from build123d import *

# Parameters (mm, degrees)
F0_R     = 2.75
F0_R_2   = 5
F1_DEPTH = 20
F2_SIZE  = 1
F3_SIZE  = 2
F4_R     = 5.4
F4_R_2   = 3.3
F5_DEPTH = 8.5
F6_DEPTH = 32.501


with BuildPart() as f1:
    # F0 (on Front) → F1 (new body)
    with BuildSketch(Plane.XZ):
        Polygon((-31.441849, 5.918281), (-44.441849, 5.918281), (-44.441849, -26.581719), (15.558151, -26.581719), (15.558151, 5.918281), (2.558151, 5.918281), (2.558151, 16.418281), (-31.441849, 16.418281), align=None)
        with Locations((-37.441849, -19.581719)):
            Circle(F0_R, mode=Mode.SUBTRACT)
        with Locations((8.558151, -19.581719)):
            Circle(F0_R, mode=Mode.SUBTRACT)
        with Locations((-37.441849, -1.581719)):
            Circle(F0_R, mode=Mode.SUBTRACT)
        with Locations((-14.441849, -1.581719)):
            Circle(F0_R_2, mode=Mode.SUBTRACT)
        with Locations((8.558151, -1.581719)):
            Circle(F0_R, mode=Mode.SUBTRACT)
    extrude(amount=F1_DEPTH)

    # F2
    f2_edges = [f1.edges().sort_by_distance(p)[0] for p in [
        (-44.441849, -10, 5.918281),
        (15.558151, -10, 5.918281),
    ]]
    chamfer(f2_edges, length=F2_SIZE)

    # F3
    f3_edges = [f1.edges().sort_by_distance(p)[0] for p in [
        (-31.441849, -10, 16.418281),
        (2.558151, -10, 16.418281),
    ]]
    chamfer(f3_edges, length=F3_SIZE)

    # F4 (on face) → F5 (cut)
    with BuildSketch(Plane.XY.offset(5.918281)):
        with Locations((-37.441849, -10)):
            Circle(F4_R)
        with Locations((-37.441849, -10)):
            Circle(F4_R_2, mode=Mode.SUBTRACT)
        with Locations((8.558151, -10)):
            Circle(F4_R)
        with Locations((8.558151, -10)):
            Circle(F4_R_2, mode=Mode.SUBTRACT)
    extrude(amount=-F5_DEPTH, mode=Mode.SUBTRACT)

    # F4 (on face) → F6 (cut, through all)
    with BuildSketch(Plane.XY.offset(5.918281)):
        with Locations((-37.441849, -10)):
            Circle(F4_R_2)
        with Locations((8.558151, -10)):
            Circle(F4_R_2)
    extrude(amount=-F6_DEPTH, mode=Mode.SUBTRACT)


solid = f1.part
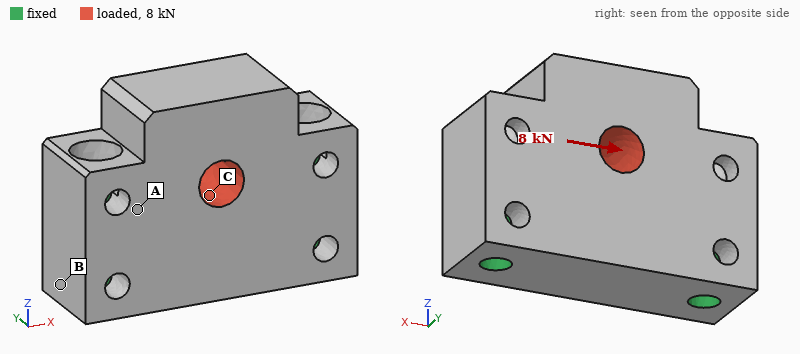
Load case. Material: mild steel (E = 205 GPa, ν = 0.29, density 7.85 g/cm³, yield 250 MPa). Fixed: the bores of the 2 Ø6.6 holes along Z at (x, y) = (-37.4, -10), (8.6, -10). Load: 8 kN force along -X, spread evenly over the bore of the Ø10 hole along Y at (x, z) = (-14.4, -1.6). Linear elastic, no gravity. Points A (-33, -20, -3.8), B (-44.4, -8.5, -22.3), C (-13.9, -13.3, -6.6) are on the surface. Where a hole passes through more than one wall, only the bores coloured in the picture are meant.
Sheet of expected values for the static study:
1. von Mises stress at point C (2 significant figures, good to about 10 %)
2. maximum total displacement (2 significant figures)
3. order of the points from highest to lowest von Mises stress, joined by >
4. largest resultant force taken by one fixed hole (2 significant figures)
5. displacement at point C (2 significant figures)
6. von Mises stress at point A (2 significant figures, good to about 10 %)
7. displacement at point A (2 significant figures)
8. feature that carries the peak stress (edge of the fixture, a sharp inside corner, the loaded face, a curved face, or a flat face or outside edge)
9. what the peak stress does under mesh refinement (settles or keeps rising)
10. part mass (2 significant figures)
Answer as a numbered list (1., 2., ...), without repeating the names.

1. 22 MPa
2. 2.2 µm
3. C > A > B
4. 4.3 kN
5. 1.2 µm
6. 11 MPa
7. 0.79 µm
8. edge of the fixture
9. keeps rising
10. 310 g
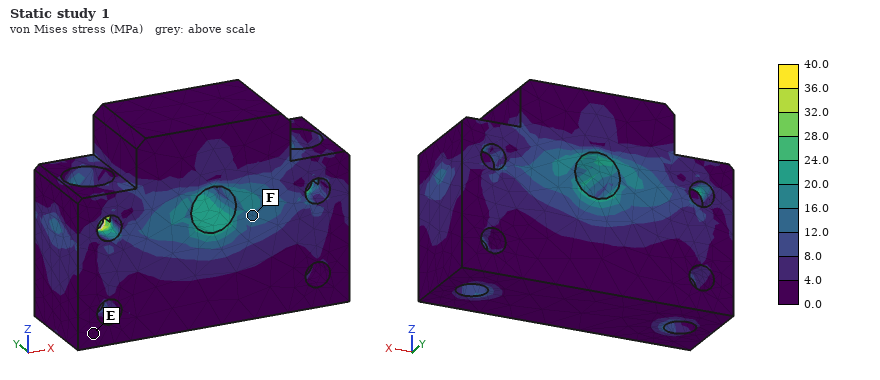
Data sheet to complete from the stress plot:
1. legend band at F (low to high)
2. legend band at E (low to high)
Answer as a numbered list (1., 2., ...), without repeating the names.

1. 12.0 to 16.0 MPa
2. 0.0 to 4.0 MPa
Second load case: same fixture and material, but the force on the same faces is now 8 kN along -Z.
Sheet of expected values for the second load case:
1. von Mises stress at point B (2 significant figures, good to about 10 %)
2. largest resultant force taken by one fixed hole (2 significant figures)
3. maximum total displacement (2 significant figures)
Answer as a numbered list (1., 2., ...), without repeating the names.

1. 4.2 MPa
2. 4.2 kN
3. 2.4 µm
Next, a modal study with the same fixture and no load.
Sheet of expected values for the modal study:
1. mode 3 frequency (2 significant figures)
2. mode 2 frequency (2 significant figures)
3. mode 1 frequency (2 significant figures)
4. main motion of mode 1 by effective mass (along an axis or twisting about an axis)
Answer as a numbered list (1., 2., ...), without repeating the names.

1. 25 kHz
2. 25 kHz
3. 12 kHz
4. along Y
